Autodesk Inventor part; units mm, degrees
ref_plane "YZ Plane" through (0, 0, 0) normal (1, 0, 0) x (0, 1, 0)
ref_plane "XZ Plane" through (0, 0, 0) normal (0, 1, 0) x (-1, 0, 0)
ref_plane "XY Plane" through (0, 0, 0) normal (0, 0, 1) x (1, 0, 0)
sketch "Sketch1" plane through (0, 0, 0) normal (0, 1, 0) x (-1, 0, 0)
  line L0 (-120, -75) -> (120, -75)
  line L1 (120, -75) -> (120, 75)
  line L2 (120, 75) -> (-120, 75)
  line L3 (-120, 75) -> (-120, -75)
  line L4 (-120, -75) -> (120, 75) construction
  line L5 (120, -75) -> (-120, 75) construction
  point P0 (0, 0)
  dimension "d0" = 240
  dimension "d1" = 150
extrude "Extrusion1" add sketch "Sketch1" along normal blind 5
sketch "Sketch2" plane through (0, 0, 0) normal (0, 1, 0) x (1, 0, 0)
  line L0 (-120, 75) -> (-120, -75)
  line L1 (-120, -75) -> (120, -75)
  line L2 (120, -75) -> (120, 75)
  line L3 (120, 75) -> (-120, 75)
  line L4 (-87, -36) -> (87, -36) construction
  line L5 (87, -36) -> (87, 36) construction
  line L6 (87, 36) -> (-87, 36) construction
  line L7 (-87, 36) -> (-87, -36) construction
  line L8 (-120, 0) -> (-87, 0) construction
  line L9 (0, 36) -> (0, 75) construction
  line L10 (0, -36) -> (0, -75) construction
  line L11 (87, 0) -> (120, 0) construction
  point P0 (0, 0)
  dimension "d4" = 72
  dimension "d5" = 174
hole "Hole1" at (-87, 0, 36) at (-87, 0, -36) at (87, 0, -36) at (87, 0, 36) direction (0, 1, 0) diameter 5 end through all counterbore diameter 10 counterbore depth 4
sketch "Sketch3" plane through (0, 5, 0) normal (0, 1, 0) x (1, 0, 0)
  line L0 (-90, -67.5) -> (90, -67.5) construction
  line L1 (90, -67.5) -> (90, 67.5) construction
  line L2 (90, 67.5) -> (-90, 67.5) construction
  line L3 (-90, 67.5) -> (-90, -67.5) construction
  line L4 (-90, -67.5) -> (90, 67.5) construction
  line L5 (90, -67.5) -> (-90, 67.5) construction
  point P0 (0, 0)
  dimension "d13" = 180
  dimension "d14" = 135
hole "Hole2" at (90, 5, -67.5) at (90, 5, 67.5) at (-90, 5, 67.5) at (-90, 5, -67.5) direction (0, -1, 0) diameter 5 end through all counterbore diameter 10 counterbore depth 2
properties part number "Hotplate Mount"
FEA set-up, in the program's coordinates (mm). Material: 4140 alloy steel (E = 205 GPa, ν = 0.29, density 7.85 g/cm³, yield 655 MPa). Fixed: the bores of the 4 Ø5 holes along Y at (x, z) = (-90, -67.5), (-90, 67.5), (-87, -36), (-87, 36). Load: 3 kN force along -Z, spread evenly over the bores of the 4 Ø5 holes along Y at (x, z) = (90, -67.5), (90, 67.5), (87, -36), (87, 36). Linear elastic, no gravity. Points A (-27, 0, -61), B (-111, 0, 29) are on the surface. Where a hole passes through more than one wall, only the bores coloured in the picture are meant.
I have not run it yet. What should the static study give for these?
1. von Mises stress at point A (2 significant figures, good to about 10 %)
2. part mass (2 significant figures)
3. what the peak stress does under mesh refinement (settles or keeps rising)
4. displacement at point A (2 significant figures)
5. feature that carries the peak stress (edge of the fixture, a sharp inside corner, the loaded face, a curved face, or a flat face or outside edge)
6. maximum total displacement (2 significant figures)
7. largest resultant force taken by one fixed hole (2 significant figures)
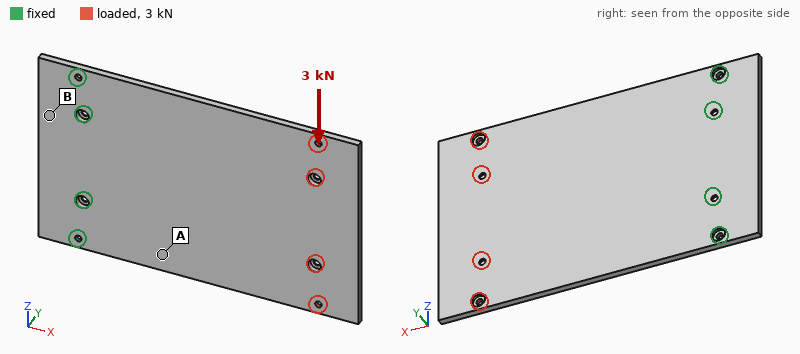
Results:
16 MPa
1.4 kg
keeps rising
15 µm
edge of the fixture
53 µm
3.4 kN
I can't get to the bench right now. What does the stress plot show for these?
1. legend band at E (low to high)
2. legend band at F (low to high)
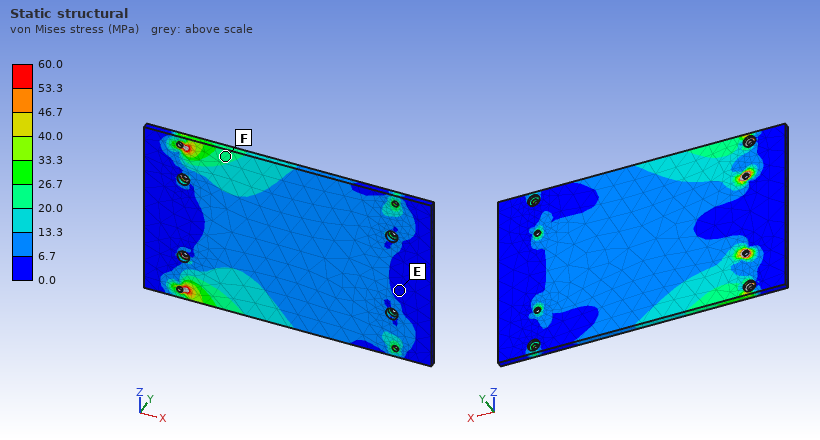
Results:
0.0 to 6.7 MPa
20.0 to 26.7 MPa
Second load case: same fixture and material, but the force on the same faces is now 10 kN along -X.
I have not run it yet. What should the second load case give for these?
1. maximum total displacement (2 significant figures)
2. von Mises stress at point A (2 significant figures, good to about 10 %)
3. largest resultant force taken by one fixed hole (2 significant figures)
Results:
0.32 mm
20 MPa
3.2 kN
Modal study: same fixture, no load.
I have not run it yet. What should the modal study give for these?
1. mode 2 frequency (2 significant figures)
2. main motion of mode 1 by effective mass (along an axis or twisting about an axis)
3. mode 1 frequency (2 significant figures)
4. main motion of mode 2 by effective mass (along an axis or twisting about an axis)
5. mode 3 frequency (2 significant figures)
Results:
300 Hz
along Y
83 Hz
twisting about X
540 Hz
